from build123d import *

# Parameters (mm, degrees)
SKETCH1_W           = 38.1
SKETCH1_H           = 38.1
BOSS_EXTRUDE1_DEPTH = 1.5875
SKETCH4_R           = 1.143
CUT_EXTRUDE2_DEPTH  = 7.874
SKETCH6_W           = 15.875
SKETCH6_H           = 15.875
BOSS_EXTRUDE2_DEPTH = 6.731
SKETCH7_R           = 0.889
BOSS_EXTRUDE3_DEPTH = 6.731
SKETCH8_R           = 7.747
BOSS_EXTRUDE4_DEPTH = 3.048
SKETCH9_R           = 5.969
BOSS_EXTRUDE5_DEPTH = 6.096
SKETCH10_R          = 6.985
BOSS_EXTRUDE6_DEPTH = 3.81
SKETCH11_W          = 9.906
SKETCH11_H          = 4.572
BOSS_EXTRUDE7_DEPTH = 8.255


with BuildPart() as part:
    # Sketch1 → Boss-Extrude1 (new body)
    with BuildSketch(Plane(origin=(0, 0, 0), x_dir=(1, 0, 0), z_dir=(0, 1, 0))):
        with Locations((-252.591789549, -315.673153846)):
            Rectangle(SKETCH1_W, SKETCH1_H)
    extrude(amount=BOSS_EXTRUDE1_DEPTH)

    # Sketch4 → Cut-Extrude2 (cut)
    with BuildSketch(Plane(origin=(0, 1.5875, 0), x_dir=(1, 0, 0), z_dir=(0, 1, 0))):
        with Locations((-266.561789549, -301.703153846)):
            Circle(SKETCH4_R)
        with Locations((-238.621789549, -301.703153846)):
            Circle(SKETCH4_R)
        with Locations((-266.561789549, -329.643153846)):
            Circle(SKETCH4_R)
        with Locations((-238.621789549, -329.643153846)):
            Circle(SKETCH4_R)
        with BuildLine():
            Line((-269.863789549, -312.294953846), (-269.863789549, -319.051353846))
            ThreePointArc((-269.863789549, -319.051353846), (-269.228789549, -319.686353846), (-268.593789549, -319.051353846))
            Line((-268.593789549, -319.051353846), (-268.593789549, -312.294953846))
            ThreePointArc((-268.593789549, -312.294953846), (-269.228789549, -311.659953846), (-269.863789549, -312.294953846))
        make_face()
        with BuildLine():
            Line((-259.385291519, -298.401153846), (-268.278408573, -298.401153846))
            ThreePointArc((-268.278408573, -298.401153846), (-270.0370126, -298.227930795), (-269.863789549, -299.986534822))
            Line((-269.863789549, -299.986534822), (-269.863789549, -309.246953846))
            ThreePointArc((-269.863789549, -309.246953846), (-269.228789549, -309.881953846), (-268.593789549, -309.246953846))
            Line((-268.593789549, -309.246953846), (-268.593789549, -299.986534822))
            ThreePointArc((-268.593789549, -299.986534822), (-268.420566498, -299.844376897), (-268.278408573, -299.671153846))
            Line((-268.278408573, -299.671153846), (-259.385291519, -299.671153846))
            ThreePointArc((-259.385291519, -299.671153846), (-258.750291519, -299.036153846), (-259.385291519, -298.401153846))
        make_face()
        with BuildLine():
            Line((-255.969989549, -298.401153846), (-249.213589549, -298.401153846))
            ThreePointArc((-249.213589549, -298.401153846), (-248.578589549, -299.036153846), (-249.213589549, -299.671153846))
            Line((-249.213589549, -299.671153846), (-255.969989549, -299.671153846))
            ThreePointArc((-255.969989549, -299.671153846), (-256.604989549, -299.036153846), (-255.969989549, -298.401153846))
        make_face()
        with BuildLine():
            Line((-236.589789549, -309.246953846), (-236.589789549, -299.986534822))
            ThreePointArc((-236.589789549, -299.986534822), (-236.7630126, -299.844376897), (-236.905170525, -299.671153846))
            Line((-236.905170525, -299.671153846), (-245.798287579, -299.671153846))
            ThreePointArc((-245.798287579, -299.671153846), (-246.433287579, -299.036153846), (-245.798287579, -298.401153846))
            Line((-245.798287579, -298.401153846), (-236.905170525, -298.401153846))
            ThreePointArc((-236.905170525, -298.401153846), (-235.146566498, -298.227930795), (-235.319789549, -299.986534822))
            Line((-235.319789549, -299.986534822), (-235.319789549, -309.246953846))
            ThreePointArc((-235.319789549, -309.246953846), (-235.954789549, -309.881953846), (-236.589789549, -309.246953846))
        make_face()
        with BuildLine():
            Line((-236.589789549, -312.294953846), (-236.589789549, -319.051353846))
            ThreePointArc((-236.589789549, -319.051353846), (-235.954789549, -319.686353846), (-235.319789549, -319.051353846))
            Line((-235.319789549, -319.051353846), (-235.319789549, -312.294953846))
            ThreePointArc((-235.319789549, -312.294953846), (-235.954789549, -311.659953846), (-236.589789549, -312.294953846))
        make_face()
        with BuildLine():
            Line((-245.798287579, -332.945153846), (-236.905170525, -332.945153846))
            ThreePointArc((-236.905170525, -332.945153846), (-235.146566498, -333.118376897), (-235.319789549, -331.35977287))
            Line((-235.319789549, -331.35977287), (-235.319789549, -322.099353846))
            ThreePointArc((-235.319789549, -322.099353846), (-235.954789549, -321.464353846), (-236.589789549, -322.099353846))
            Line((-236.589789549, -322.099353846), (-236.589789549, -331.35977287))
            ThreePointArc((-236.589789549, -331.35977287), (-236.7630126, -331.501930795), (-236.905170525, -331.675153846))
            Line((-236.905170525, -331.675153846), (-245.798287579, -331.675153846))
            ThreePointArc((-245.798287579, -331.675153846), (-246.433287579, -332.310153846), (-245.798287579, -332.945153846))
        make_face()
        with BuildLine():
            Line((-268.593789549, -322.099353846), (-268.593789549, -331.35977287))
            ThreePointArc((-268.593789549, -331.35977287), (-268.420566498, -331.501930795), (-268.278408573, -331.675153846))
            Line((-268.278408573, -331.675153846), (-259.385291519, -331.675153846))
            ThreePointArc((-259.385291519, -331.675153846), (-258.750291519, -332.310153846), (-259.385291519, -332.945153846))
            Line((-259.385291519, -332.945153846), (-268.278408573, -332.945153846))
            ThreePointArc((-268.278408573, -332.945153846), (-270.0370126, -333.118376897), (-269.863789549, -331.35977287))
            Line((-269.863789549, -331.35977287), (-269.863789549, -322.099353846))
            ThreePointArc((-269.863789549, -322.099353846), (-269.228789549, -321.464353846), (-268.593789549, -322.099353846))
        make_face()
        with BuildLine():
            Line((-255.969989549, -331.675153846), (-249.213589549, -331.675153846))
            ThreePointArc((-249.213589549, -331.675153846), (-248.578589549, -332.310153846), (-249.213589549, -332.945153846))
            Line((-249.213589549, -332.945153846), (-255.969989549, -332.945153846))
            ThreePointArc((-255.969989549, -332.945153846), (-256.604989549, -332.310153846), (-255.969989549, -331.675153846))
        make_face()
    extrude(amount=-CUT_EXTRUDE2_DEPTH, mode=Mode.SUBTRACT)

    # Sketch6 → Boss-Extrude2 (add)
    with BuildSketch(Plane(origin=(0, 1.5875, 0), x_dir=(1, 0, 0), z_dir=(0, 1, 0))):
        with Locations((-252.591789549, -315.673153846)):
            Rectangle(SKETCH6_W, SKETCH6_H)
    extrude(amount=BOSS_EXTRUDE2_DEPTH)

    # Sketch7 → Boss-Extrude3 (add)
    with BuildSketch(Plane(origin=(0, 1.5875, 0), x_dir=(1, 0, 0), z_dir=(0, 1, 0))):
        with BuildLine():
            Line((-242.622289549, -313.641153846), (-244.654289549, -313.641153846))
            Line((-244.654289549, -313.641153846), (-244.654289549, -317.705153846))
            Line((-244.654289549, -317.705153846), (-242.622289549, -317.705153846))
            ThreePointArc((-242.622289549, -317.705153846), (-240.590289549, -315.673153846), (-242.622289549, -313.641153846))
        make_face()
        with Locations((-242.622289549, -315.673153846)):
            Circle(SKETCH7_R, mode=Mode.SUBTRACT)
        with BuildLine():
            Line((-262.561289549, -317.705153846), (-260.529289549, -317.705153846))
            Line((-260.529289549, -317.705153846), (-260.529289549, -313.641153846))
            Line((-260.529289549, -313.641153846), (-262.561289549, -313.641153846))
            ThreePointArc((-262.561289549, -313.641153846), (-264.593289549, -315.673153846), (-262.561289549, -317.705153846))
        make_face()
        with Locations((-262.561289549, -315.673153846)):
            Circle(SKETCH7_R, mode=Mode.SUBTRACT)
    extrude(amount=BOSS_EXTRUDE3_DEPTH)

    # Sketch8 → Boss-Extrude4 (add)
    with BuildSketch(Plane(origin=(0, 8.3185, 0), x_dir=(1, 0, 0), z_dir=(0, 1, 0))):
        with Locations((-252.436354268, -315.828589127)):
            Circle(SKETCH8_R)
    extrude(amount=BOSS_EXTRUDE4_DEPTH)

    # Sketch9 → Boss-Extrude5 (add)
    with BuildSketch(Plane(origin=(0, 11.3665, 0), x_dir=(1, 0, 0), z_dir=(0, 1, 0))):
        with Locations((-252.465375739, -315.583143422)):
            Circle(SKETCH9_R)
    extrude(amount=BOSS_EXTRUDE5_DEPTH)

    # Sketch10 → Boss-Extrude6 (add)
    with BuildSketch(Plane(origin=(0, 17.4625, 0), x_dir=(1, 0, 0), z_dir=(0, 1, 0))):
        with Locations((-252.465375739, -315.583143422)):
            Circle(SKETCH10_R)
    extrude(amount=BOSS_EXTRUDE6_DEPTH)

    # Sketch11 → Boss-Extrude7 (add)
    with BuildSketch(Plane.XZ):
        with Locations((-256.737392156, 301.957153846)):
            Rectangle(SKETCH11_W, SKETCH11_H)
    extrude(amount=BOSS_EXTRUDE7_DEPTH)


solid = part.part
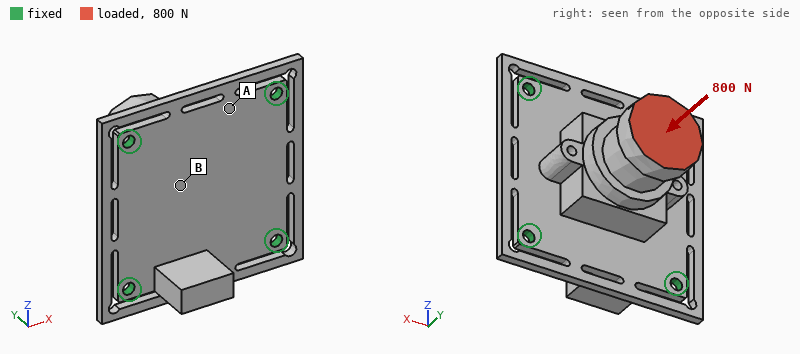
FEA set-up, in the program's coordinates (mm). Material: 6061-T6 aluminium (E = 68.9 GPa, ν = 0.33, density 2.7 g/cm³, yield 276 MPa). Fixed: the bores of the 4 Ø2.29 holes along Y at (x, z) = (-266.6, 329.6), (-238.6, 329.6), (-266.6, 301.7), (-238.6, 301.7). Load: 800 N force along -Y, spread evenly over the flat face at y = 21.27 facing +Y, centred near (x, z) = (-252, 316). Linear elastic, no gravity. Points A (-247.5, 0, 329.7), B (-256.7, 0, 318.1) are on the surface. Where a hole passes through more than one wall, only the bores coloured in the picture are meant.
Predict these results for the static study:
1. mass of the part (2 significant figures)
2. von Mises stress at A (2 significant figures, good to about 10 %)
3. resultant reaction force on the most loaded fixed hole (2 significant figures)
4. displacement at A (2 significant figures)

17 g
48 MPa
220 N
42 µm
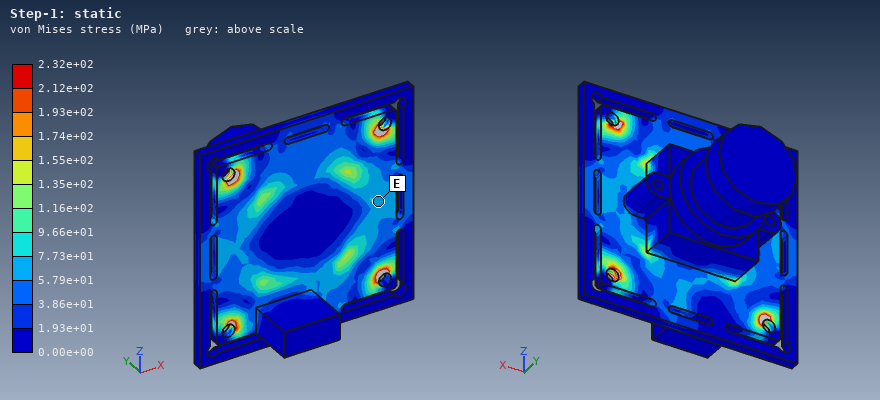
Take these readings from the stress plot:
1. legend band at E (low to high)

5.79e+01 to 7.73e+01 MPa
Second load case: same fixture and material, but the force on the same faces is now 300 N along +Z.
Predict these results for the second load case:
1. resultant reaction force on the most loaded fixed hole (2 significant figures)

160 N
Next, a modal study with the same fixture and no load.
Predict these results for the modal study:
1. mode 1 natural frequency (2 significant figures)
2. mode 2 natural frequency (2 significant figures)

4700 Hz
4800 Hz
